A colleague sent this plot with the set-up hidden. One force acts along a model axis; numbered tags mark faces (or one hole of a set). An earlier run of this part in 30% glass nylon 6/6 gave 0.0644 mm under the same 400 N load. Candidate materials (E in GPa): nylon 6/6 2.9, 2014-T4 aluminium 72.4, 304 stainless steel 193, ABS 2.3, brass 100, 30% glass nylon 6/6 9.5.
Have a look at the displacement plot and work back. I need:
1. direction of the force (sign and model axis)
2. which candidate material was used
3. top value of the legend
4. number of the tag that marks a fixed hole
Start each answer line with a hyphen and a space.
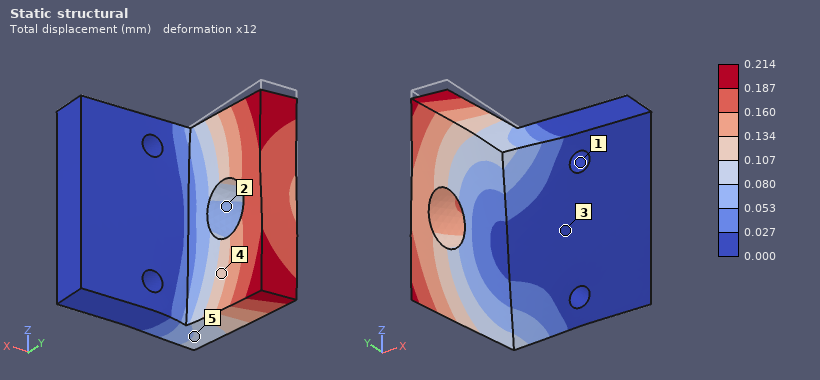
- -Z
- nylon 6/6
- 0.214 mm
- 1
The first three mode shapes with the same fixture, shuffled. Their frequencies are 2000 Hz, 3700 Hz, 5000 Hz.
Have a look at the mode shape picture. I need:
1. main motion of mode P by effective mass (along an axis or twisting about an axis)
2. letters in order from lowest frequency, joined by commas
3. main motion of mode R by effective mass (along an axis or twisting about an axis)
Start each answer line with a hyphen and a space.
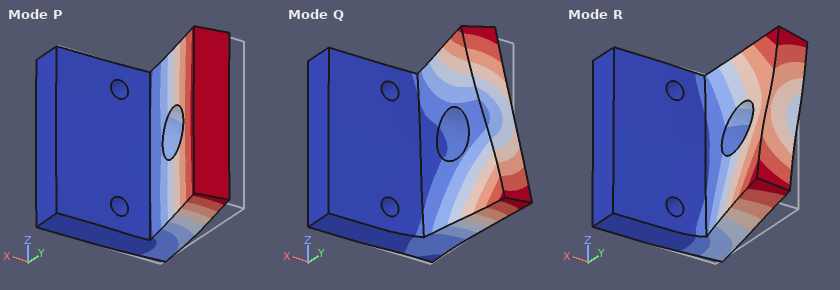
- along X
- P, R, Q
- along Z
